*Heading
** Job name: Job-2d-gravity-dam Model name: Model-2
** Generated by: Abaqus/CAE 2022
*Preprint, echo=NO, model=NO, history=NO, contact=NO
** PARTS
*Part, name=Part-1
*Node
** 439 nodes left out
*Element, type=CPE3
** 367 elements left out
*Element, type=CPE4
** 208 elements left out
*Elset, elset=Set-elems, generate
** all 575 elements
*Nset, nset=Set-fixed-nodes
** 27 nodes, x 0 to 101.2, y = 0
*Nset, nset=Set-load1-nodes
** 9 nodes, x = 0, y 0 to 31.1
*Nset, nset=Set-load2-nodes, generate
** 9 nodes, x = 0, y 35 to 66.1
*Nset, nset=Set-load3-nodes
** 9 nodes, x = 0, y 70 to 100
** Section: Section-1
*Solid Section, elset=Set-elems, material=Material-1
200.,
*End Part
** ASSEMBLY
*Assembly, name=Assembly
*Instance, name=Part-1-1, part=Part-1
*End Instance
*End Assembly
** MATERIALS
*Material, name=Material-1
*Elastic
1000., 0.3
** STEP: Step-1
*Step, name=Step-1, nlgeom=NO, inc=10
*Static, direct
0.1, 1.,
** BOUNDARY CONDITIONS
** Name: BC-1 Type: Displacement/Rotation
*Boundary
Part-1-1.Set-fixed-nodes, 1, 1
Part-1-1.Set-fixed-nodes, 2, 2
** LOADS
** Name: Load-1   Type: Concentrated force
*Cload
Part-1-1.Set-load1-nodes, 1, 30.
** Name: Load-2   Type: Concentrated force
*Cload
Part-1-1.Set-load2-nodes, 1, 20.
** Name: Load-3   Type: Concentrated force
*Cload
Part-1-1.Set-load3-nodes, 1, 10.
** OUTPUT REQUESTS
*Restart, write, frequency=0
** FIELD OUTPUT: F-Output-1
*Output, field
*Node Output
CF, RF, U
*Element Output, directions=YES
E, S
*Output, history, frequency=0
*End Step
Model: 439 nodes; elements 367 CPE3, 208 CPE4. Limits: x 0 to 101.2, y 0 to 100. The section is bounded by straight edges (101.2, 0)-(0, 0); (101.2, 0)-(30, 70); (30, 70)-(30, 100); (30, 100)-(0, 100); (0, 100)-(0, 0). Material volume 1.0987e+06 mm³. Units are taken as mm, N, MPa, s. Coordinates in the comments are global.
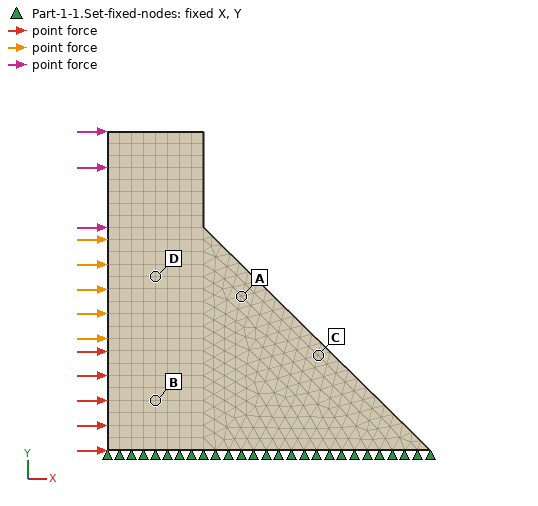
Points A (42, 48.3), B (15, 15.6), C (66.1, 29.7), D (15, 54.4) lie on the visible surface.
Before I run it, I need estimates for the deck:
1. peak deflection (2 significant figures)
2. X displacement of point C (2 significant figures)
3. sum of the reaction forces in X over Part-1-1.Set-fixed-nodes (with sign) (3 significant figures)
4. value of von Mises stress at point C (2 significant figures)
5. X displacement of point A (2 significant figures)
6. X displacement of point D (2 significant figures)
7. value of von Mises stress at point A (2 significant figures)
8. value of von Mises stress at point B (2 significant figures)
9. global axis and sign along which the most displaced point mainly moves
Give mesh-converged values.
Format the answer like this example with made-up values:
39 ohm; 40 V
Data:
0.016 mm; 0.0021 mm; -540 N; 0.061 MPa; 0.0047 mm; 0.0062 mm; 0.057 MPa; 0.072 MPa; +X
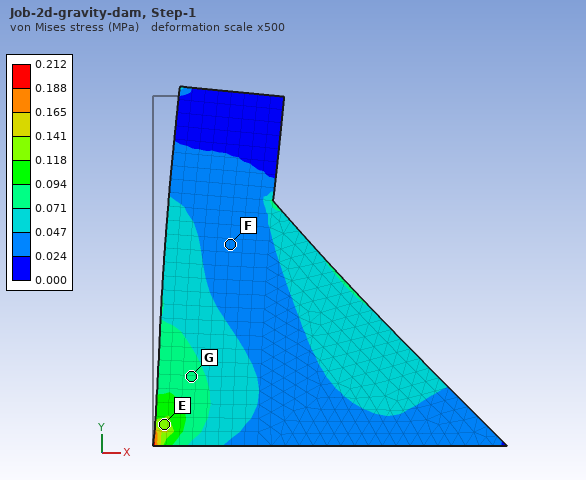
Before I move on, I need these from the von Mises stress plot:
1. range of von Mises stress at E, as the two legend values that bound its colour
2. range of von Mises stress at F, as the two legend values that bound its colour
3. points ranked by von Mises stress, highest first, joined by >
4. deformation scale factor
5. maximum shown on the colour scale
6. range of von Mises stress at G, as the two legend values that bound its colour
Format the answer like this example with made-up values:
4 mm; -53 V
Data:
0.118 to 0.141 MPa; 0.024 to 0.047 MPa; E > G > F; 500; 0.212 MPa; 0.071 to 0.094 MPa
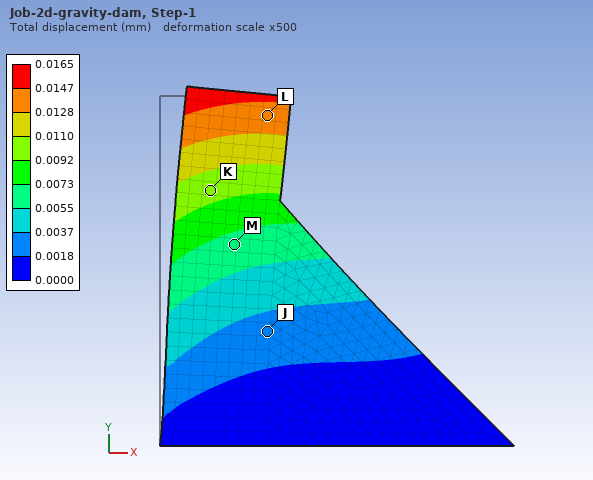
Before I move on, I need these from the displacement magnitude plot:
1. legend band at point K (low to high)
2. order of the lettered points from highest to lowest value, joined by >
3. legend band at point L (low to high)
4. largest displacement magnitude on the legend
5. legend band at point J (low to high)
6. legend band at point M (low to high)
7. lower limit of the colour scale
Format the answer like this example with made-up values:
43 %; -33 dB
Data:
0.0092 to 0.0110 mm; L > K > M > J; 0.0128 to 0.0147 mm; 0.0165 mm; 0.0018 to 0.0037 mm; 0.0055 to 0.0073 mm; 0.0000 mm
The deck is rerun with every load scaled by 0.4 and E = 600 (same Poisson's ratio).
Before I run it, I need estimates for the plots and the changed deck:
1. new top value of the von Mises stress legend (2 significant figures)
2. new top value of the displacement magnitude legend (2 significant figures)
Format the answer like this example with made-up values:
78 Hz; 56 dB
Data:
0.085 MPa; 0.011 mm
